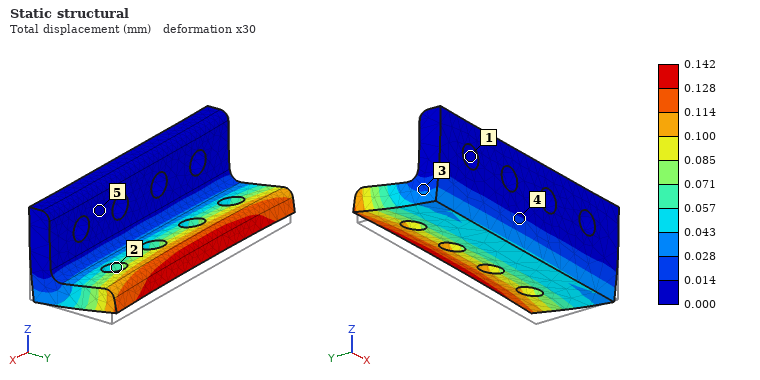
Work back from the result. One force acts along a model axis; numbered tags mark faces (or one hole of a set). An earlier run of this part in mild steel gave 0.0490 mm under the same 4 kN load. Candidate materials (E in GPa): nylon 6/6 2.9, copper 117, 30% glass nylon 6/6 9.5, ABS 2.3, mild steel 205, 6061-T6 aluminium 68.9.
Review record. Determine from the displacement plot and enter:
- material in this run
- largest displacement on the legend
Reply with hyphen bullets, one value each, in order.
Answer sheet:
- 6061-T6 aluminium
- 0.142 mm
